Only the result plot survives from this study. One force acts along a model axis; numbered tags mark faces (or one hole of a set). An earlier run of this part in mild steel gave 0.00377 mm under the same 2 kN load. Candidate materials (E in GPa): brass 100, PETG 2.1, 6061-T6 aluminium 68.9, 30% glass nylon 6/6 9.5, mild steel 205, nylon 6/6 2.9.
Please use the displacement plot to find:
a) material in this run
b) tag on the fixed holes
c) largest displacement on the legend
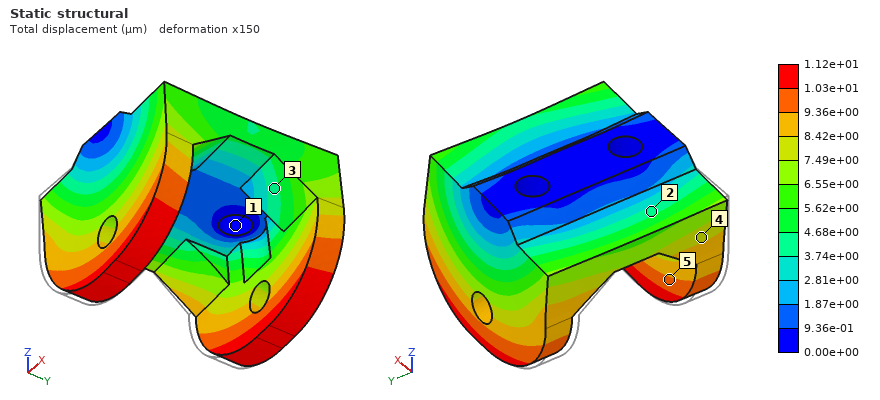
6061-T6 aluminium
1
1.12e+01 µm
